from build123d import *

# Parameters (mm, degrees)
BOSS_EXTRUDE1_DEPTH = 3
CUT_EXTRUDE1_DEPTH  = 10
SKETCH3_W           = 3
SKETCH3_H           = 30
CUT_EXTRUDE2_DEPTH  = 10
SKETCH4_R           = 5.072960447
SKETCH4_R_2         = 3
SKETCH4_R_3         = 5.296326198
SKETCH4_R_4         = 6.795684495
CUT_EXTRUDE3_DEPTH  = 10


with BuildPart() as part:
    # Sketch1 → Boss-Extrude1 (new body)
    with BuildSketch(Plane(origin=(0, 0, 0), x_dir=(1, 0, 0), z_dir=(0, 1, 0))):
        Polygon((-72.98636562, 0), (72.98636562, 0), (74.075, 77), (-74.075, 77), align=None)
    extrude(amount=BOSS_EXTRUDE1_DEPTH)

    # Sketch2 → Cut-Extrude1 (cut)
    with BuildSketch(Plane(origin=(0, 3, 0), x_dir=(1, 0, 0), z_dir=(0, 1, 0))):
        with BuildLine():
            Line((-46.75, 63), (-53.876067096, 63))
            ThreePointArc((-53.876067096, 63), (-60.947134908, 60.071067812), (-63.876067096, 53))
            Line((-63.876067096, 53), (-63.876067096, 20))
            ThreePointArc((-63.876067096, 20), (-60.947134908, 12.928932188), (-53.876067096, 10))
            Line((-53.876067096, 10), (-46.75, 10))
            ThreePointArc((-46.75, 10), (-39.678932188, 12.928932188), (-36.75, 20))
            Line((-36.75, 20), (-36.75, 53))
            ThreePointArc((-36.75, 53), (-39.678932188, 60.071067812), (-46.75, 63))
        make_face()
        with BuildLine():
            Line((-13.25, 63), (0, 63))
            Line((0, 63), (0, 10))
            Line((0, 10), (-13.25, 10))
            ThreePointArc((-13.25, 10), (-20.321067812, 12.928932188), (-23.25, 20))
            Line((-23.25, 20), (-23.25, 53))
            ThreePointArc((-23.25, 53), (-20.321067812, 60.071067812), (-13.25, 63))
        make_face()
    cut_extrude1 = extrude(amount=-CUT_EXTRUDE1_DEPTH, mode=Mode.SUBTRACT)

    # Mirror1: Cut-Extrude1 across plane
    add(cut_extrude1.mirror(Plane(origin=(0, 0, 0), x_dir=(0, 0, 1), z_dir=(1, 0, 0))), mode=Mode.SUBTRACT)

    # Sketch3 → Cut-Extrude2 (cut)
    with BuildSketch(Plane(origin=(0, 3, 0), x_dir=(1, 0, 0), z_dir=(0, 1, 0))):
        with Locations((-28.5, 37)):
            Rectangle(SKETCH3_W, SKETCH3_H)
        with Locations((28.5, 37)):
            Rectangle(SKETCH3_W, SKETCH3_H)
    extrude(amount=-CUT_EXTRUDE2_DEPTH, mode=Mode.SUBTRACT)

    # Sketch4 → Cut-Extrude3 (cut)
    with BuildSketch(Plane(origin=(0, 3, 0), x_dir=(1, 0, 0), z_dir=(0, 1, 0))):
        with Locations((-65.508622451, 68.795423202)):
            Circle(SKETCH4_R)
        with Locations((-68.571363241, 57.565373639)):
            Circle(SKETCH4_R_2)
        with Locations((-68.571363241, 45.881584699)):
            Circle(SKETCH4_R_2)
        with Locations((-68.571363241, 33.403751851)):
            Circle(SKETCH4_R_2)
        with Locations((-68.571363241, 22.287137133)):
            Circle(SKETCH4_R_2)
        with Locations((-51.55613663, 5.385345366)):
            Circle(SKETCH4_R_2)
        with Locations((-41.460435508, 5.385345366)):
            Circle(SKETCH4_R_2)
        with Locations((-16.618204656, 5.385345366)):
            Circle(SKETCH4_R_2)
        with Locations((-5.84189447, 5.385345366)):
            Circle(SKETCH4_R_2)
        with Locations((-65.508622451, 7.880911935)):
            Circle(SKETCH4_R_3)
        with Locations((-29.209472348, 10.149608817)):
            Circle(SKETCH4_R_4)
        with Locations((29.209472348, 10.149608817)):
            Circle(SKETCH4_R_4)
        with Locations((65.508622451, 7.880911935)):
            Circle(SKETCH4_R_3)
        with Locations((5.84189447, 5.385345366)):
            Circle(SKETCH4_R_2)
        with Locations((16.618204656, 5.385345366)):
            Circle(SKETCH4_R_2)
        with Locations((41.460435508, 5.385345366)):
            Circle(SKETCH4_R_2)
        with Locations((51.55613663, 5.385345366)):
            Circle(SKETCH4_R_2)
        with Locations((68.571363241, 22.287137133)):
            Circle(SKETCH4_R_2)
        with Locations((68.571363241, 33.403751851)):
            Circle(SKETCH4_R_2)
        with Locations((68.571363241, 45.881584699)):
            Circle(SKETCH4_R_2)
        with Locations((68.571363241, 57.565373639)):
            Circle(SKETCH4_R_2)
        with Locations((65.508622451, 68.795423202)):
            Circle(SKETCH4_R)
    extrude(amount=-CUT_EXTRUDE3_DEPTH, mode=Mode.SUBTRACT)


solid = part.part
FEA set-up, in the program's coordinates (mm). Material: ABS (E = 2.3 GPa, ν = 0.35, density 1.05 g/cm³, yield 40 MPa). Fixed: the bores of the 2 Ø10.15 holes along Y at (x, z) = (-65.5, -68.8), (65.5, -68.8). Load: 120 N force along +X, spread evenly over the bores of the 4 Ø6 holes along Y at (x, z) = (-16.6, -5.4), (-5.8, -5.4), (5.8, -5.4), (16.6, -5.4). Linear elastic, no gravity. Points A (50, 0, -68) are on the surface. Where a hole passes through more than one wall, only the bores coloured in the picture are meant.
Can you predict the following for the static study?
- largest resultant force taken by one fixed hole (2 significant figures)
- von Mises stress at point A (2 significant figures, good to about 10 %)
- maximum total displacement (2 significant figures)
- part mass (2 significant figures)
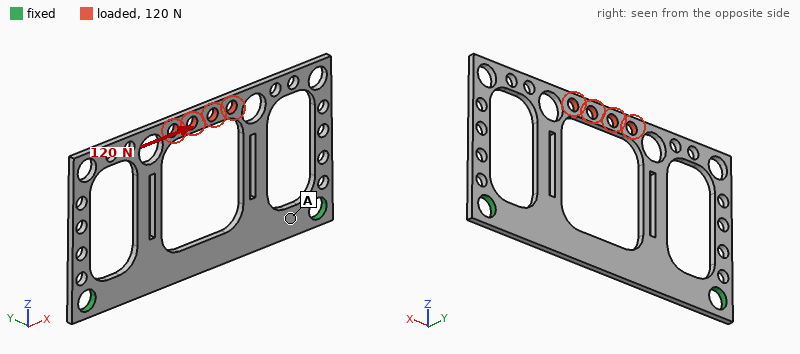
76 N
1.6 MPa
1.2 mm
16 g
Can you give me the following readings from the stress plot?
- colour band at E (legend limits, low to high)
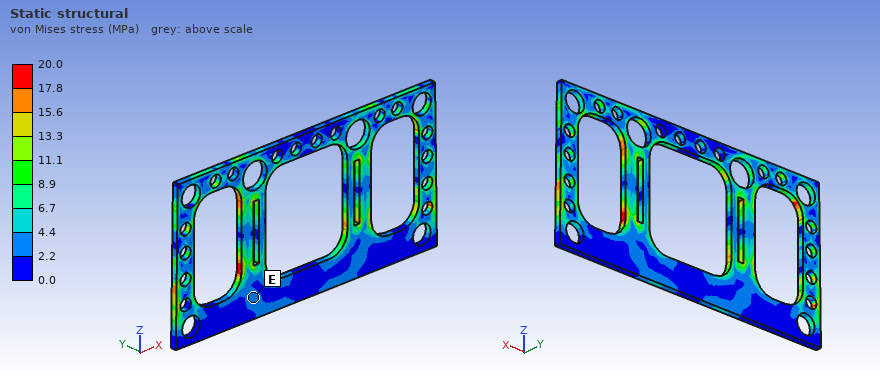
2.2 to 4.4 MPa
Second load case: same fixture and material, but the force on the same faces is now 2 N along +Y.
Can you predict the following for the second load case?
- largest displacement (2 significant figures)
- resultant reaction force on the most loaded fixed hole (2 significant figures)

1.7 mm
1.0 N
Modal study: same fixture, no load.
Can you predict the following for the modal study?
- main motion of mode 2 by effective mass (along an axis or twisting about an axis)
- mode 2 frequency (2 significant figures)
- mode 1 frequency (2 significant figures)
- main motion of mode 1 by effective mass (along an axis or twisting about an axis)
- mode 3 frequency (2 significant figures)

twisting about Z
170 Hz
99 Hz
along Y
260 Hz
